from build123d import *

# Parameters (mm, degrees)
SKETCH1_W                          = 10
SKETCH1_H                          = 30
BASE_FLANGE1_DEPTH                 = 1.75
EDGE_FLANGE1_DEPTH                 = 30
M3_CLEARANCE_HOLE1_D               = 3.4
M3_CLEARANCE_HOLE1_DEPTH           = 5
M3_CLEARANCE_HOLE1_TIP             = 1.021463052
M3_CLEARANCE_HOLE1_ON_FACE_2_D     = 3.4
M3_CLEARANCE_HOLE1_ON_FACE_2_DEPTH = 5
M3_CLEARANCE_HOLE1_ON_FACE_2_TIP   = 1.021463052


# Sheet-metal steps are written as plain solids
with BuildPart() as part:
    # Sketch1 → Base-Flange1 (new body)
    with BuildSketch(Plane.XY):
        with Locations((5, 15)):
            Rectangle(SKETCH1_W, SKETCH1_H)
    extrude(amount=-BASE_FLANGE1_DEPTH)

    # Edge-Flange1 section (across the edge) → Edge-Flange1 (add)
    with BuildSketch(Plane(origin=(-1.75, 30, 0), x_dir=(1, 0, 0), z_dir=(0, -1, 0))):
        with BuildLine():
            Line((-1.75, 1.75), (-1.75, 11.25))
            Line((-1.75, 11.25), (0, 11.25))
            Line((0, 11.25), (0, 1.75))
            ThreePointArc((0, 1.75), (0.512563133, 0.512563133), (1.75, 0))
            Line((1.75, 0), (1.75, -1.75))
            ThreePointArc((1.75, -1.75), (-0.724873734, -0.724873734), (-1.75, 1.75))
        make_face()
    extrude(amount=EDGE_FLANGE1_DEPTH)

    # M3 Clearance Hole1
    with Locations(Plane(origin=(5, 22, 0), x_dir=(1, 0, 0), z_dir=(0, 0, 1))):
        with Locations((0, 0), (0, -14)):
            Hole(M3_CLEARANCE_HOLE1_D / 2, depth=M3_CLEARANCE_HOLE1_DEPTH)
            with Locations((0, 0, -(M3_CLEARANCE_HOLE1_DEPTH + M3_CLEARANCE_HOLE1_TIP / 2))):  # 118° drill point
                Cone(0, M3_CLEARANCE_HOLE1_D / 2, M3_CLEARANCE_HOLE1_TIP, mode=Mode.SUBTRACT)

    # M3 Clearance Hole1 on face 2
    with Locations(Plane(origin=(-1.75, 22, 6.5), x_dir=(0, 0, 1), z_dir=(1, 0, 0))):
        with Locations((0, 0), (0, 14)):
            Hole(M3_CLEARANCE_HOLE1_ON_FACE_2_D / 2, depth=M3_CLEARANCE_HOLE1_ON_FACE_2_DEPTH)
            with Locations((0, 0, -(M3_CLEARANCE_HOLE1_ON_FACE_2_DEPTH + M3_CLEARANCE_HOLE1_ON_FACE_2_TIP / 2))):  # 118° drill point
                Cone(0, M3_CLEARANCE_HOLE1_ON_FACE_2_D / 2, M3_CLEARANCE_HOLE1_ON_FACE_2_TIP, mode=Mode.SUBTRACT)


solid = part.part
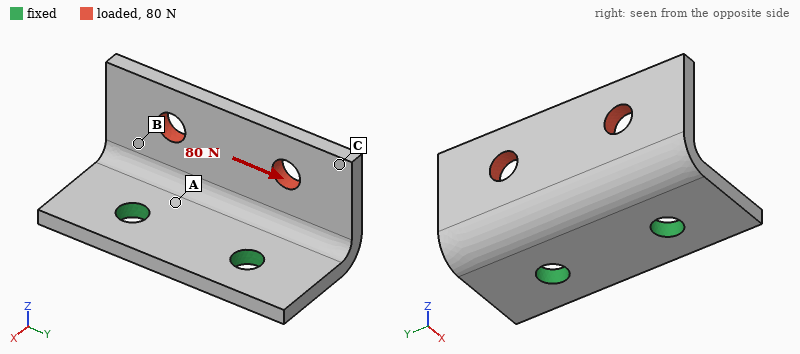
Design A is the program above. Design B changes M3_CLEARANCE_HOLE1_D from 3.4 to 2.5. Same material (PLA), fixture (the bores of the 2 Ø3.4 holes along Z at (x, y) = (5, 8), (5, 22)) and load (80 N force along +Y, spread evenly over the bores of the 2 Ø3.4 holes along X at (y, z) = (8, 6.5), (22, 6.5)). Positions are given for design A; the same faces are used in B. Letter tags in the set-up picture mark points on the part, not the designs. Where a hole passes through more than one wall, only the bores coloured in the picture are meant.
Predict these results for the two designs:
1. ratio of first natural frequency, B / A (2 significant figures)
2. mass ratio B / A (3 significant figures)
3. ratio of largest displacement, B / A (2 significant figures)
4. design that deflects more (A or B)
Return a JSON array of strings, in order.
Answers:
["0.94", "1.01", "1.2", "B"]
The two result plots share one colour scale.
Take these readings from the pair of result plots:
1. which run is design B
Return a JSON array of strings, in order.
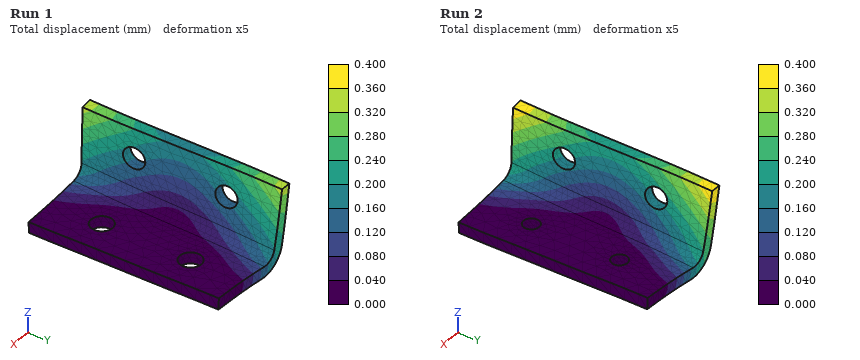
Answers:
["Run 2"]
